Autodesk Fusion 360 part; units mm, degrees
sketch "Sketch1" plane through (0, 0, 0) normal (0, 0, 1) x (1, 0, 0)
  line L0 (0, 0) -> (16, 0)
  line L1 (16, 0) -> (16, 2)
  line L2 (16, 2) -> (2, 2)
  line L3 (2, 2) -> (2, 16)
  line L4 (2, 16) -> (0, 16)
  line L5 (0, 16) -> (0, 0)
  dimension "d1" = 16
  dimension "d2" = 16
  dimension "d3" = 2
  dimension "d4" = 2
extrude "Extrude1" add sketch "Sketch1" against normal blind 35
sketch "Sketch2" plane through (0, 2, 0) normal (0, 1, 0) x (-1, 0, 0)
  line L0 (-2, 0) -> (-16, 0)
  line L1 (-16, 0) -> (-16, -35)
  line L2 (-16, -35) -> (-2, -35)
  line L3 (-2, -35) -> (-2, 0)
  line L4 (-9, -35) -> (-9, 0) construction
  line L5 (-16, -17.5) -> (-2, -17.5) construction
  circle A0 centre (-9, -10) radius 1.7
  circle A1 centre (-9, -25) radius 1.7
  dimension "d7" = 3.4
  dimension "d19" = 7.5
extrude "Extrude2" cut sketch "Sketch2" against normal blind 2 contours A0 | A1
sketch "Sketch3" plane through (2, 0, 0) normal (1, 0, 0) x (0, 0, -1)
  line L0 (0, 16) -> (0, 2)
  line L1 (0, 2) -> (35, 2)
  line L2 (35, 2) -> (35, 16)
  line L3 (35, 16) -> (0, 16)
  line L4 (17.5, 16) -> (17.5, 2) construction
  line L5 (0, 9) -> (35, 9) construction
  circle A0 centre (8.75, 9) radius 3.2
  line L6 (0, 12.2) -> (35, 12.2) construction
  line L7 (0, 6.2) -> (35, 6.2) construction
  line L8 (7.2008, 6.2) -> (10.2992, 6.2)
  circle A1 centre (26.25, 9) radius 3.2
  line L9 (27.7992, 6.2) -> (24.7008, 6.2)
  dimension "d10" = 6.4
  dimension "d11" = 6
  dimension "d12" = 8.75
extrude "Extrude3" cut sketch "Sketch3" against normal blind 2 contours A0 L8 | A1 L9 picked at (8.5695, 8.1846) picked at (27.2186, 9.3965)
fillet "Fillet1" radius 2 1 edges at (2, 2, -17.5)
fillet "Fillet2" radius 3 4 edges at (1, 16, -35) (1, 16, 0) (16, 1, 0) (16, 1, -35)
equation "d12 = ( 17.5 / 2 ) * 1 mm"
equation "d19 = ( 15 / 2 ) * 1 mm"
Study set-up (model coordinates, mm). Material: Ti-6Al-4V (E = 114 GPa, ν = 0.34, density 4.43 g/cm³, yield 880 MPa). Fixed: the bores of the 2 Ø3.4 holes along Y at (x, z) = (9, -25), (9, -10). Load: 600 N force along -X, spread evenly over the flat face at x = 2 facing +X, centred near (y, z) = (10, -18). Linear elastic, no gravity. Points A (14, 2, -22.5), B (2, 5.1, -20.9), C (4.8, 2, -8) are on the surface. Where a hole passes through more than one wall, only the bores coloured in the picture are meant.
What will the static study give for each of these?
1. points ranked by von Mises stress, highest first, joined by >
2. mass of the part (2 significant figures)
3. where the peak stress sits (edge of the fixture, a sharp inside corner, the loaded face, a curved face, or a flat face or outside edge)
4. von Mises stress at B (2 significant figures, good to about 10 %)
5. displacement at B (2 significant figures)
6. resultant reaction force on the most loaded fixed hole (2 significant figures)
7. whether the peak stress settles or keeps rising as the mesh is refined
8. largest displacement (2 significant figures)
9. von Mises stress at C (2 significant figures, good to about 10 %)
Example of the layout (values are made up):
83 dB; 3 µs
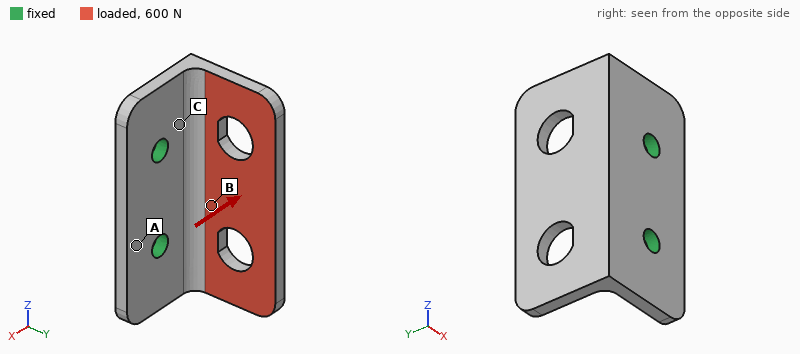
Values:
C > B > A; 8.7 g; edge of the fixture; 150 MPa; 0.072 mm; 300 N; keeps rising; 0.30 mm; 240 MPa
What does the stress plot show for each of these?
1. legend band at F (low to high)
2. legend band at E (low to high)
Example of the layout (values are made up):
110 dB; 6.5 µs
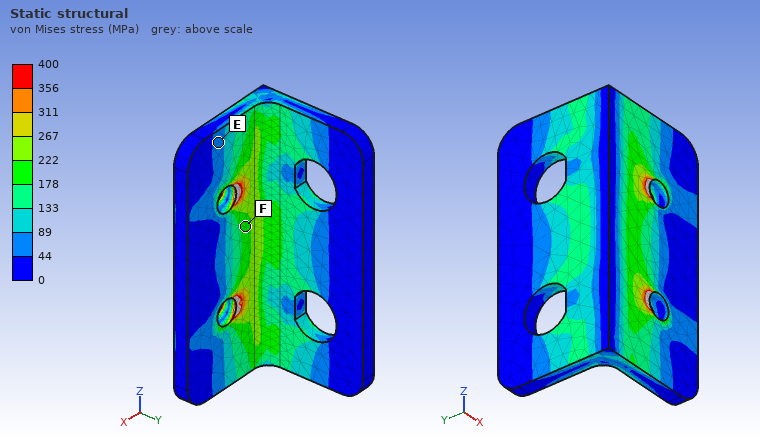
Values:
178 to 222 MPa; 44 to 89 MPa
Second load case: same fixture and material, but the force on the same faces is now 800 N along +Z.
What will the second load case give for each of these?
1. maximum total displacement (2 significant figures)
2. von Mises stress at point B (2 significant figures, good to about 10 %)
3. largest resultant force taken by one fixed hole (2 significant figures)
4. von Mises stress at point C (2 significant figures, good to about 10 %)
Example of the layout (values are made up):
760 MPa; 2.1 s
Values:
0.10 mm; 92 MPa; 630 N; 83 MPa
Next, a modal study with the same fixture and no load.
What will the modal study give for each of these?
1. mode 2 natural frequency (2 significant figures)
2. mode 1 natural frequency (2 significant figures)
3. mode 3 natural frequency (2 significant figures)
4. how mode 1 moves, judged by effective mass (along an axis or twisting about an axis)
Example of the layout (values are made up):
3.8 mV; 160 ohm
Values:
6800 Hz; 4600 Hz; 11 kHz; along X
